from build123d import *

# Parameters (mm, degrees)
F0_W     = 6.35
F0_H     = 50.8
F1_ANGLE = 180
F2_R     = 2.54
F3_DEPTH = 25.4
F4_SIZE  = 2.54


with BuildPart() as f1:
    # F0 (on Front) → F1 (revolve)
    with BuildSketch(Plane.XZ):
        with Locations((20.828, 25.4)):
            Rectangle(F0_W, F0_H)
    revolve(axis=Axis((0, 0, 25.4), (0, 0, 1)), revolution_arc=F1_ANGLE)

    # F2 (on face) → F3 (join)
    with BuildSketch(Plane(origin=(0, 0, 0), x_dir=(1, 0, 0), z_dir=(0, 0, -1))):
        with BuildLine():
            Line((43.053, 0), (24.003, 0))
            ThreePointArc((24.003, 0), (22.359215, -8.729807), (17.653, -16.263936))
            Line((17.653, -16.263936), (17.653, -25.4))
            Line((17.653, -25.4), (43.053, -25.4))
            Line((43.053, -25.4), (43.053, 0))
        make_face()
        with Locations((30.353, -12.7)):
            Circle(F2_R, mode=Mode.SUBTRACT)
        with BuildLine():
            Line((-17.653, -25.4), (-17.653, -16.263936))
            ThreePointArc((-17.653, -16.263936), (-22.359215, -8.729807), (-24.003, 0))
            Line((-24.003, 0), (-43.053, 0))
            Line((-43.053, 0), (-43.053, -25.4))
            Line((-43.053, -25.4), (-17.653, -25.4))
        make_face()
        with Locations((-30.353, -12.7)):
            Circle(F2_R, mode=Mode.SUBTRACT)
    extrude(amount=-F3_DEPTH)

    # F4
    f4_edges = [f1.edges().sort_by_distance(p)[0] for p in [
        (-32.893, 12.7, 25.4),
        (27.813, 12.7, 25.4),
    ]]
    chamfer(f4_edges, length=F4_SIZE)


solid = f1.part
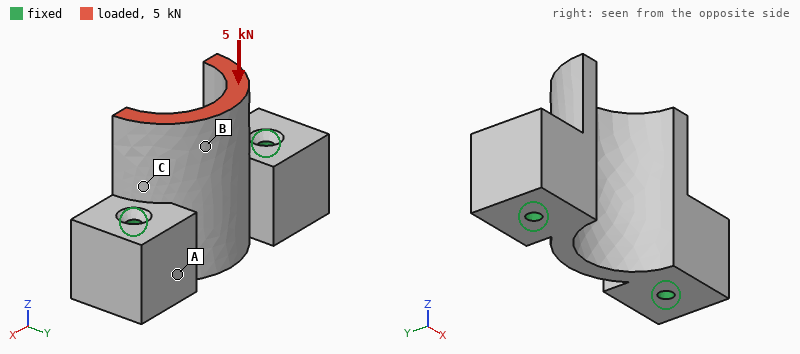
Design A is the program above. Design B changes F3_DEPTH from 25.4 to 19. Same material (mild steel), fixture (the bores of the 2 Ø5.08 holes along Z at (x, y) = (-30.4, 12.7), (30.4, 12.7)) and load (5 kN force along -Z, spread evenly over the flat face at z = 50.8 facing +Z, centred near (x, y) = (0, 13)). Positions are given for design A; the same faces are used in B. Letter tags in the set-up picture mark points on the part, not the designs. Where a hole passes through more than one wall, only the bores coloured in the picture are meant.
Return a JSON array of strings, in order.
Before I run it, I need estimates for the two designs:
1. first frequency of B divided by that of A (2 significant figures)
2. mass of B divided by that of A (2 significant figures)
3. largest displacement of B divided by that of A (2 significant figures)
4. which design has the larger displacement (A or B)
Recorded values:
["0.72", "0.86", "1.5", "B"]
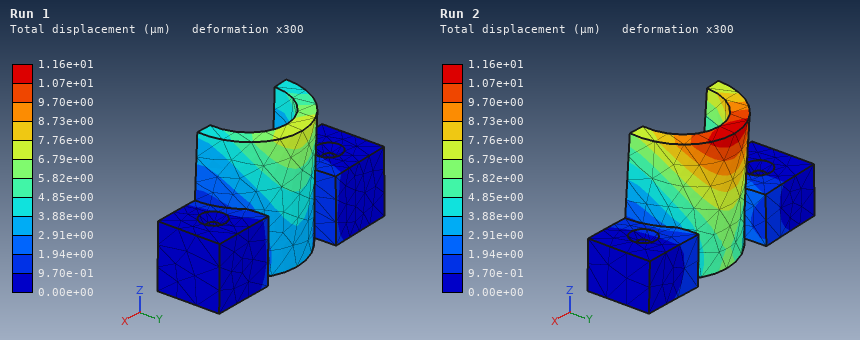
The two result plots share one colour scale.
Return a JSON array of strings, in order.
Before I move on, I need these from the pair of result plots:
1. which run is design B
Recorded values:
["Run 2"]
